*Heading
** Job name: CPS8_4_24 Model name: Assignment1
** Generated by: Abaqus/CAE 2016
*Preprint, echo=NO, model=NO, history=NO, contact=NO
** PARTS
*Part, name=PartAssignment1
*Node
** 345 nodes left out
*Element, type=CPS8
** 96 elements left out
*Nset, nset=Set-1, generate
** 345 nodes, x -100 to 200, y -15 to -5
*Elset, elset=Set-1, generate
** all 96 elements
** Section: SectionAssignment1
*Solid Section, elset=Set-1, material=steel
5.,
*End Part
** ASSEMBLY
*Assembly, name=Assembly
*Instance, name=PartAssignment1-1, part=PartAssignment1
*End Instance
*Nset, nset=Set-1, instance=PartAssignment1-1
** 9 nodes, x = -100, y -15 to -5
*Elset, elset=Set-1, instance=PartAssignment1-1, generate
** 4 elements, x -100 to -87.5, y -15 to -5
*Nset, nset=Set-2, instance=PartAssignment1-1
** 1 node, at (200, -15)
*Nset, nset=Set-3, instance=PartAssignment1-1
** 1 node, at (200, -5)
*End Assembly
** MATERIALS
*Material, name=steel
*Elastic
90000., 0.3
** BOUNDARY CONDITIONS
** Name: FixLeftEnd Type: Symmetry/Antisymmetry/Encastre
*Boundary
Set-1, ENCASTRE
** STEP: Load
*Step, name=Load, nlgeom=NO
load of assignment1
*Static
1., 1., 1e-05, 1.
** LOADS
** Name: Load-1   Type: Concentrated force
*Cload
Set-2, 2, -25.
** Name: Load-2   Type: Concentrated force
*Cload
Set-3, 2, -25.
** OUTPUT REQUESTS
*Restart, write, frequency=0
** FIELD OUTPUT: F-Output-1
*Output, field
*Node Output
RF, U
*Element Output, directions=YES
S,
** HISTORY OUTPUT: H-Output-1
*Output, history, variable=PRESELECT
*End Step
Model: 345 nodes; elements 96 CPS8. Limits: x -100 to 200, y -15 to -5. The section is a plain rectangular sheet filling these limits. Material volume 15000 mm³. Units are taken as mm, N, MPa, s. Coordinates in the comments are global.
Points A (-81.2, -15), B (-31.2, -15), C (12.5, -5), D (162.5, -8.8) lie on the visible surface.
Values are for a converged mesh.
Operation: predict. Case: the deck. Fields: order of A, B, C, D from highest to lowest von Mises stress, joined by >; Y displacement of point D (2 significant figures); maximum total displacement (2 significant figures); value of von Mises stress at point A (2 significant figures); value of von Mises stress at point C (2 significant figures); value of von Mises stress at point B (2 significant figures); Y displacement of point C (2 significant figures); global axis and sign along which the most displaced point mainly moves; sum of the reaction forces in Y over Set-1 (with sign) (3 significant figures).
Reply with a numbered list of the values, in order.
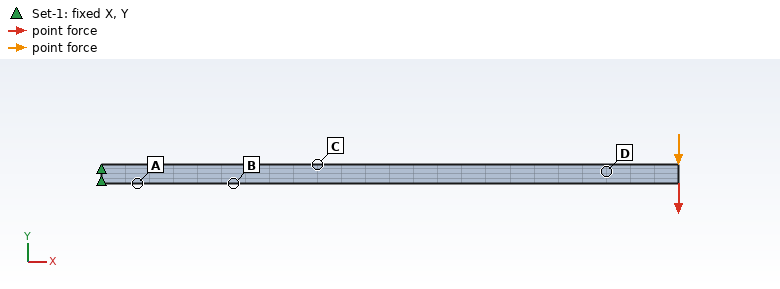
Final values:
1. A > B > C > D
2. -9.7 mm
3. 12 mm
4. 170 MPa
5. 110 MPa
6. 140 MPa
7. -2.2 mm
8. -Y
9. 50.0 N
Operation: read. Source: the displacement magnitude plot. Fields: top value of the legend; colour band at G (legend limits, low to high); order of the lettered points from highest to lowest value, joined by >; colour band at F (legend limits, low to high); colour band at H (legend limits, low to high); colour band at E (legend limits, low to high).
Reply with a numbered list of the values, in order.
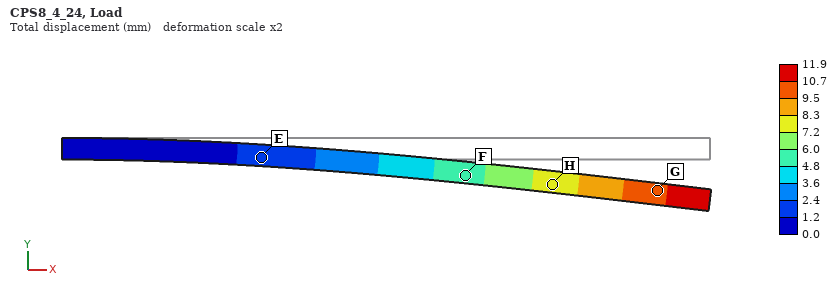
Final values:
1. 11.9 mm
2. 9.5 to 10.7 mm
3. G > H > F > E
4. 4.8 to 6.0 mm
5. 7.2 to 8.3 mm
6. 1.2 to 2.4 mm
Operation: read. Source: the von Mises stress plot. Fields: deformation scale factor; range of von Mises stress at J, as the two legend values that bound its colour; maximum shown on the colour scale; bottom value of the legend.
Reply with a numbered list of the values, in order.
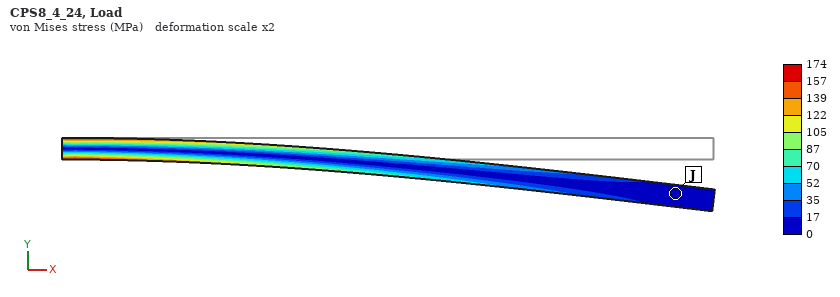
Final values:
1. 2
2. 0 to 17 MPa
3. 174 MPa
4. 0 MPa
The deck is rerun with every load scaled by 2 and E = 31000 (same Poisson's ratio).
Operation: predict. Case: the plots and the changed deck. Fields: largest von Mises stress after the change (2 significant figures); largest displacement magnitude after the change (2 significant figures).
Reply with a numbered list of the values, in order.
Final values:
1. 350 MPa
2. 69 mm
